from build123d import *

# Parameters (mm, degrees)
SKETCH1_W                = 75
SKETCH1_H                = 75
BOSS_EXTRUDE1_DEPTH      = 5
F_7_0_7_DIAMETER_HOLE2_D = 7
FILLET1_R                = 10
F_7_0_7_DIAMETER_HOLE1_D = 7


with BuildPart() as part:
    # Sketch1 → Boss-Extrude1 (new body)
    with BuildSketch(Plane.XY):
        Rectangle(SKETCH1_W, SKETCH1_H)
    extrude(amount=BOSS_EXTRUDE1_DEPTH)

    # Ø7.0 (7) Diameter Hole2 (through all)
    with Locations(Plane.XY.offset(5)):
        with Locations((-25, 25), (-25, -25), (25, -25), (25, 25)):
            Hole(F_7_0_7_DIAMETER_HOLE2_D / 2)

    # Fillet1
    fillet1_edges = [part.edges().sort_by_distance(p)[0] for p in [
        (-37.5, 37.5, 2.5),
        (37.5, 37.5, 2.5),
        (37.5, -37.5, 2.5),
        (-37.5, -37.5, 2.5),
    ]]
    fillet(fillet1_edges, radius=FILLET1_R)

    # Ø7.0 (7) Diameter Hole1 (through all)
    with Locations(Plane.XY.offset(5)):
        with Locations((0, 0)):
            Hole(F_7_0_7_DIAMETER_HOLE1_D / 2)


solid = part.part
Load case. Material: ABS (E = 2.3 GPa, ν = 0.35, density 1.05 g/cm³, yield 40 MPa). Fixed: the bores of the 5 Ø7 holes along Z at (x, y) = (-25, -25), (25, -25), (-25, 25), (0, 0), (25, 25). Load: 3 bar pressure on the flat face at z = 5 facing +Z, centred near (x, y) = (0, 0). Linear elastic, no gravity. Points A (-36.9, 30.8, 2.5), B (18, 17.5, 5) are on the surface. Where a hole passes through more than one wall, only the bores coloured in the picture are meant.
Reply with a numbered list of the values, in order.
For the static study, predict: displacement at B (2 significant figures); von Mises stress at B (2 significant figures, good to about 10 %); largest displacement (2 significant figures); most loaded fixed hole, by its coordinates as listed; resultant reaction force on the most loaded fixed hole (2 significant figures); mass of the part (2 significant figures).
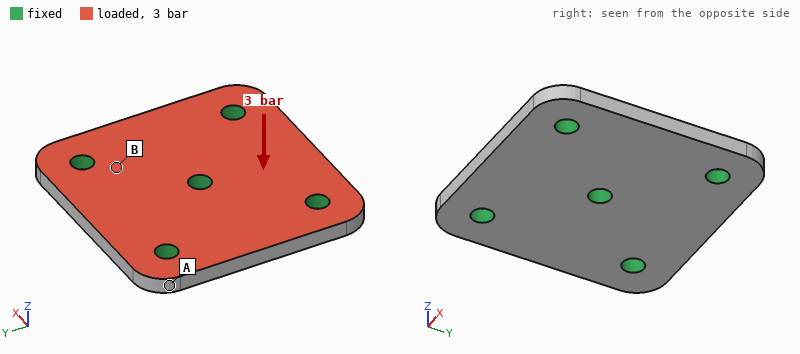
1. 0.042 mm
2. 5.3 MPa
3. 0.20 mm
4. (0, 0)
5. 360 N
6. 28 g
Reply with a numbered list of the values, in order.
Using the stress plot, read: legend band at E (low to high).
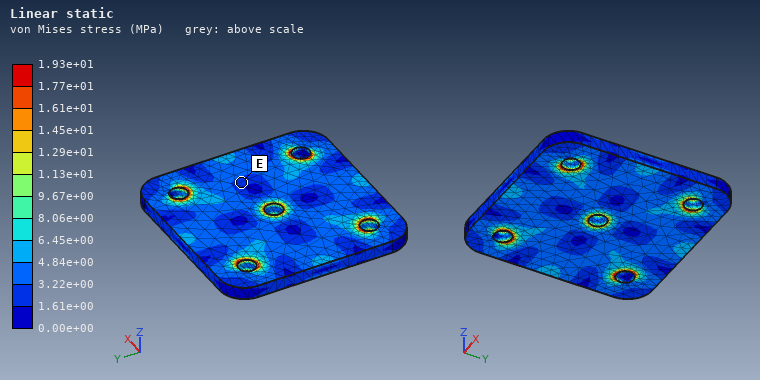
1. 1.61e+00 to 3.22e+00 MPa
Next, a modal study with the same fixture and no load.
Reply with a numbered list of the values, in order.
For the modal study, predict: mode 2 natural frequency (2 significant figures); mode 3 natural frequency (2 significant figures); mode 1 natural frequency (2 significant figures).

1. 3400 Hz
2. 3400 Hz
3. 3300 Hz
